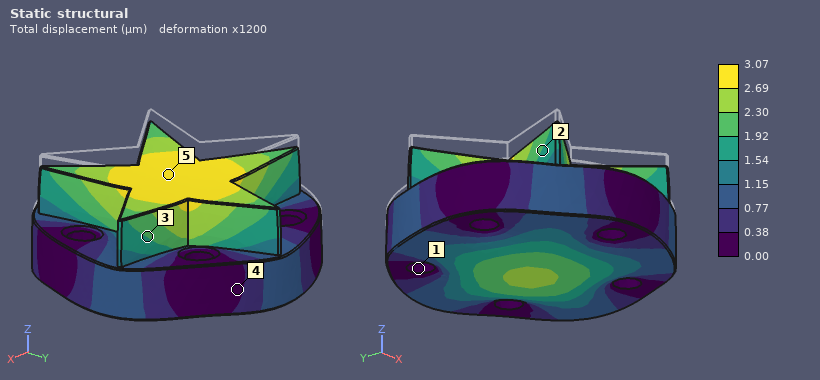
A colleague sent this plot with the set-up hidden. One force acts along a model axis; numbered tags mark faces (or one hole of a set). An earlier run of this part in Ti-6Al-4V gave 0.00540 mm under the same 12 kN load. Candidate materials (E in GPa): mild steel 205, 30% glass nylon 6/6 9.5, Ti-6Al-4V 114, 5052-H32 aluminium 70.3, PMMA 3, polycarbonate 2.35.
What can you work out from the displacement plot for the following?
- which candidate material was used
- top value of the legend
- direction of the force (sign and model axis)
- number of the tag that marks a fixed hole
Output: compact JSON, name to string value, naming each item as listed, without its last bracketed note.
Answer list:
{"which candidate material was used": "mild steel", "top value of the legend": "3.07 µm", "direction of the force": "-Z", "number of the tag that marks a fixed hole": "1"}
